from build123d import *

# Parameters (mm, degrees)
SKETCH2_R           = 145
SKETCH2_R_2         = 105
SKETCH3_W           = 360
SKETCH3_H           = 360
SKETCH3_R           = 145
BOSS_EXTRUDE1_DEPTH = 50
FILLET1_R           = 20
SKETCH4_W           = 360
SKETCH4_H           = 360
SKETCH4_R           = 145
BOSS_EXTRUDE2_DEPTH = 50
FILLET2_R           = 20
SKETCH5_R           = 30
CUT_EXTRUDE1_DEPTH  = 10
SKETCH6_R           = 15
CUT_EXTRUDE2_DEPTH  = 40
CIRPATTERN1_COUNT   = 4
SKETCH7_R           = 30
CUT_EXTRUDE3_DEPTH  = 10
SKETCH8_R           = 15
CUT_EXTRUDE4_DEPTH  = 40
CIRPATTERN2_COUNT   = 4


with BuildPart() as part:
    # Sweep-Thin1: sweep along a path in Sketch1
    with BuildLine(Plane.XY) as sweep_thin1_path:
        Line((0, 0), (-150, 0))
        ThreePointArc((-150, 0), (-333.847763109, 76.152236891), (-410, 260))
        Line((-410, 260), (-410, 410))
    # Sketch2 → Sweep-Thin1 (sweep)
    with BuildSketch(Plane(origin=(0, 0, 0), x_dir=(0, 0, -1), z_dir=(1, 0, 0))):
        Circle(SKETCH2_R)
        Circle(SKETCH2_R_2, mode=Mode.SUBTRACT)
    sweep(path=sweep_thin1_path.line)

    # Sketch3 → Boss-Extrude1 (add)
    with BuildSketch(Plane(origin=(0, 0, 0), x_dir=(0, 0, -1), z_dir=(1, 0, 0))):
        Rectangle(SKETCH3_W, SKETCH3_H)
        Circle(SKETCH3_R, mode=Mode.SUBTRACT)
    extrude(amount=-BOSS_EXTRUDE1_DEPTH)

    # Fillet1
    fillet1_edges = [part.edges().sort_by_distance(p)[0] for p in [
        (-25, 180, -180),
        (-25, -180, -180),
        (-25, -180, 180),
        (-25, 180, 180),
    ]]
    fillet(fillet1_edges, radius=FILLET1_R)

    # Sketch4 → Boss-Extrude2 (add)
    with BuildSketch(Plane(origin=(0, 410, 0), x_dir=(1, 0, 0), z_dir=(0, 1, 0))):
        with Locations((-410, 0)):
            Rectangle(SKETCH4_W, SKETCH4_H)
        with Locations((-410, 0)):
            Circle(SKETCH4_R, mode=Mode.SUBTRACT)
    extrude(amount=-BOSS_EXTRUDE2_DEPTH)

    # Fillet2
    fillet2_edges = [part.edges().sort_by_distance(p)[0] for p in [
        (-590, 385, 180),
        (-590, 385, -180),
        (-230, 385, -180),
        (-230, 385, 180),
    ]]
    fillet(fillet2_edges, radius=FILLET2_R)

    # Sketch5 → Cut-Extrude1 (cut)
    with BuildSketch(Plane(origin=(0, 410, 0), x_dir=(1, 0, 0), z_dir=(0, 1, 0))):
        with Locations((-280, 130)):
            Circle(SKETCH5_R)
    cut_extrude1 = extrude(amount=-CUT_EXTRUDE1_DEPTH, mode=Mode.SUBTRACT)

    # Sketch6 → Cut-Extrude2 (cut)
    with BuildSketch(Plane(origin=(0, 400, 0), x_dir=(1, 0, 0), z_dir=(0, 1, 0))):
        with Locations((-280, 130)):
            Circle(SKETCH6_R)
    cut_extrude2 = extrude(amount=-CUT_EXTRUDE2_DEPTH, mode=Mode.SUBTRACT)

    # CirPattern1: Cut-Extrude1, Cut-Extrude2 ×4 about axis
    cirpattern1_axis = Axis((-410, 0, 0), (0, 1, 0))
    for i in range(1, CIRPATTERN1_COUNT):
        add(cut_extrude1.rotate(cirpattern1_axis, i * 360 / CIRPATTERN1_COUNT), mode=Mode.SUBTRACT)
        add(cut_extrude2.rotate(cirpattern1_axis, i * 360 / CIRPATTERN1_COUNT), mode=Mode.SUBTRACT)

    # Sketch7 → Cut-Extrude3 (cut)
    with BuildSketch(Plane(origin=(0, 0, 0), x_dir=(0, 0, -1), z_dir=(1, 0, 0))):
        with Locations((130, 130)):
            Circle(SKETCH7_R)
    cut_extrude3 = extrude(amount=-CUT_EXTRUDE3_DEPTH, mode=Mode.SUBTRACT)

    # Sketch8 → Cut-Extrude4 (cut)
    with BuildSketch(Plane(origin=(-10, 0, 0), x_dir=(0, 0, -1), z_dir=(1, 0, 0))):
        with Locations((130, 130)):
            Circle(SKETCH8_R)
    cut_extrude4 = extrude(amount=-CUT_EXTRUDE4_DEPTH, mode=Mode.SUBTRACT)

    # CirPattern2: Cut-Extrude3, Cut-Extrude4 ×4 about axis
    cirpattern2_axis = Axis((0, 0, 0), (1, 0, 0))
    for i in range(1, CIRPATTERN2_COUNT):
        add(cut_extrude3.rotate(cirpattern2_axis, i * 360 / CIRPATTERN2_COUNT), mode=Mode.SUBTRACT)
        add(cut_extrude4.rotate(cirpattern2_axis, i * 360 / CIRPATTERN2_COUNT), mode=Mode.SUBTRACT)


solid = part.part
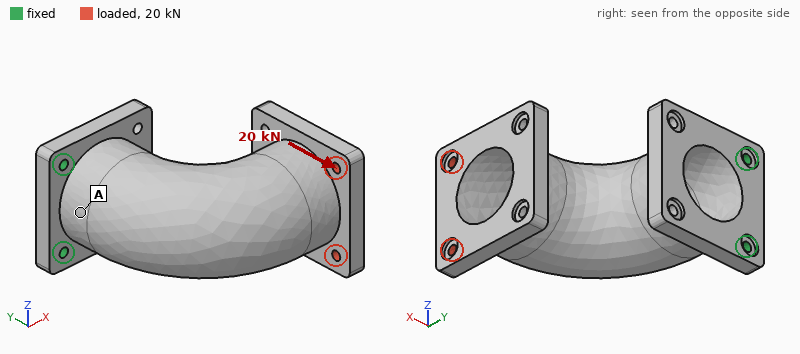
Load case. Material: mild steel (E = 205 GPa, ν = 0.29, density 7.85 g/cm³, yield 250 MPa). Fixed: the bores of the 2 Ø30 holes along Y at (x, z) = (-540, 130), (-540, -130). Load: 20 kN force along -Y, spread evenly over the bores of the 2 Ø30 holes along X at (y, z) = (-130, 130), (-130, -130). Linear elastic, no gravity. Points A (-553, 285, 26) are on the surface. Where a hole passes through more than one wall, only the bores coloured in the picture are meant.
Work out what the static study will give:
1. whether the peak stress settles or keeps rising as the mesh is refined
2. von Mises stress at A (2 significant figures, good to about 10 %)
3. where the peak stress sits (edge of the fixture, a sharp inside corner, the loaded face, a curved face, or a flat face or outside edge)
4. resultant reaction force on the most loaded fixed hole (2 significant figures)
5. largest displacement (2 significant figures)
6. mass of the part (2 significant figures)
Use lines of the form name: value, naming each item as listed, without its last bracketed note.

whether the peak stress settles or keeps rising as the mesh is refined: keeps rising
von Mises stress at A: 12 MPa
where the peak stress sits: edge of the fixture
resultant reaction force on the most loaded fixed hole: 10 kN
largest displacement: 1.0 mm
mass of the part: 220 kg
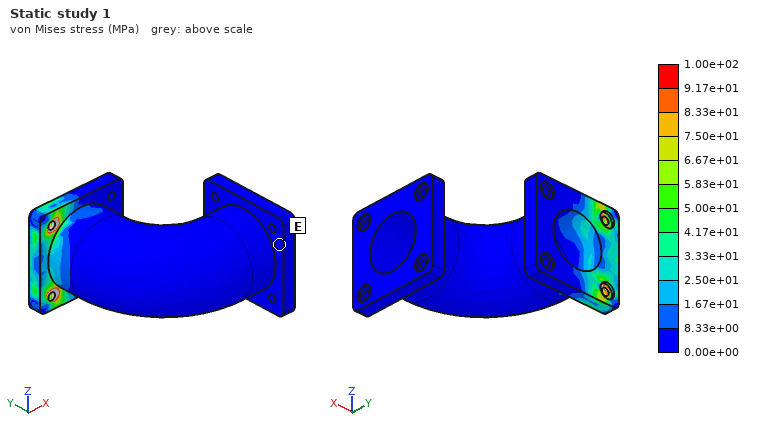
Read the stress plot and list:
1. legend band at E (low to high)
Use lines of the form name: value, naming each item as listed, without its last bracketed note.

legend band at E: 0.00e+00 to 8.33e+00 MPa
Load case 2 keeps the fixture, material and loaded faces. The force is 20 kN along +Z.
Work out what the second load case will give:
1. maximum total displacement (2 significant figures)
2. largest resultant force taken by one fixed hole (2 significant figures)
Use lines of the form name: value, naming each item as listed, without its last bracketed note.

maximum total displacement: 0.17 mm
largest resultant force taken by one fixed hole: 56 kN
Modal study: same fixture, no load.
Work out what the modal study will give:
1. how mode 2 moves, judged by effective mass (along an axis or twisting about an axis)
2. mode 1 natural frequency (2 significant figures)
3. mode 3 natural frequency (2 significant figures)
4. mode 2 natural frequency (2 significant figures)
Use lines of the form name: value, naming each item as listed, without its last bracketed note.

how mode 2 moves, judged by effective mass: along Z
mode 1 natural frequency: 69 Hz
mode 3 natural frequency: 550 Hz
mode 2 natural frequency: 220 Hz
